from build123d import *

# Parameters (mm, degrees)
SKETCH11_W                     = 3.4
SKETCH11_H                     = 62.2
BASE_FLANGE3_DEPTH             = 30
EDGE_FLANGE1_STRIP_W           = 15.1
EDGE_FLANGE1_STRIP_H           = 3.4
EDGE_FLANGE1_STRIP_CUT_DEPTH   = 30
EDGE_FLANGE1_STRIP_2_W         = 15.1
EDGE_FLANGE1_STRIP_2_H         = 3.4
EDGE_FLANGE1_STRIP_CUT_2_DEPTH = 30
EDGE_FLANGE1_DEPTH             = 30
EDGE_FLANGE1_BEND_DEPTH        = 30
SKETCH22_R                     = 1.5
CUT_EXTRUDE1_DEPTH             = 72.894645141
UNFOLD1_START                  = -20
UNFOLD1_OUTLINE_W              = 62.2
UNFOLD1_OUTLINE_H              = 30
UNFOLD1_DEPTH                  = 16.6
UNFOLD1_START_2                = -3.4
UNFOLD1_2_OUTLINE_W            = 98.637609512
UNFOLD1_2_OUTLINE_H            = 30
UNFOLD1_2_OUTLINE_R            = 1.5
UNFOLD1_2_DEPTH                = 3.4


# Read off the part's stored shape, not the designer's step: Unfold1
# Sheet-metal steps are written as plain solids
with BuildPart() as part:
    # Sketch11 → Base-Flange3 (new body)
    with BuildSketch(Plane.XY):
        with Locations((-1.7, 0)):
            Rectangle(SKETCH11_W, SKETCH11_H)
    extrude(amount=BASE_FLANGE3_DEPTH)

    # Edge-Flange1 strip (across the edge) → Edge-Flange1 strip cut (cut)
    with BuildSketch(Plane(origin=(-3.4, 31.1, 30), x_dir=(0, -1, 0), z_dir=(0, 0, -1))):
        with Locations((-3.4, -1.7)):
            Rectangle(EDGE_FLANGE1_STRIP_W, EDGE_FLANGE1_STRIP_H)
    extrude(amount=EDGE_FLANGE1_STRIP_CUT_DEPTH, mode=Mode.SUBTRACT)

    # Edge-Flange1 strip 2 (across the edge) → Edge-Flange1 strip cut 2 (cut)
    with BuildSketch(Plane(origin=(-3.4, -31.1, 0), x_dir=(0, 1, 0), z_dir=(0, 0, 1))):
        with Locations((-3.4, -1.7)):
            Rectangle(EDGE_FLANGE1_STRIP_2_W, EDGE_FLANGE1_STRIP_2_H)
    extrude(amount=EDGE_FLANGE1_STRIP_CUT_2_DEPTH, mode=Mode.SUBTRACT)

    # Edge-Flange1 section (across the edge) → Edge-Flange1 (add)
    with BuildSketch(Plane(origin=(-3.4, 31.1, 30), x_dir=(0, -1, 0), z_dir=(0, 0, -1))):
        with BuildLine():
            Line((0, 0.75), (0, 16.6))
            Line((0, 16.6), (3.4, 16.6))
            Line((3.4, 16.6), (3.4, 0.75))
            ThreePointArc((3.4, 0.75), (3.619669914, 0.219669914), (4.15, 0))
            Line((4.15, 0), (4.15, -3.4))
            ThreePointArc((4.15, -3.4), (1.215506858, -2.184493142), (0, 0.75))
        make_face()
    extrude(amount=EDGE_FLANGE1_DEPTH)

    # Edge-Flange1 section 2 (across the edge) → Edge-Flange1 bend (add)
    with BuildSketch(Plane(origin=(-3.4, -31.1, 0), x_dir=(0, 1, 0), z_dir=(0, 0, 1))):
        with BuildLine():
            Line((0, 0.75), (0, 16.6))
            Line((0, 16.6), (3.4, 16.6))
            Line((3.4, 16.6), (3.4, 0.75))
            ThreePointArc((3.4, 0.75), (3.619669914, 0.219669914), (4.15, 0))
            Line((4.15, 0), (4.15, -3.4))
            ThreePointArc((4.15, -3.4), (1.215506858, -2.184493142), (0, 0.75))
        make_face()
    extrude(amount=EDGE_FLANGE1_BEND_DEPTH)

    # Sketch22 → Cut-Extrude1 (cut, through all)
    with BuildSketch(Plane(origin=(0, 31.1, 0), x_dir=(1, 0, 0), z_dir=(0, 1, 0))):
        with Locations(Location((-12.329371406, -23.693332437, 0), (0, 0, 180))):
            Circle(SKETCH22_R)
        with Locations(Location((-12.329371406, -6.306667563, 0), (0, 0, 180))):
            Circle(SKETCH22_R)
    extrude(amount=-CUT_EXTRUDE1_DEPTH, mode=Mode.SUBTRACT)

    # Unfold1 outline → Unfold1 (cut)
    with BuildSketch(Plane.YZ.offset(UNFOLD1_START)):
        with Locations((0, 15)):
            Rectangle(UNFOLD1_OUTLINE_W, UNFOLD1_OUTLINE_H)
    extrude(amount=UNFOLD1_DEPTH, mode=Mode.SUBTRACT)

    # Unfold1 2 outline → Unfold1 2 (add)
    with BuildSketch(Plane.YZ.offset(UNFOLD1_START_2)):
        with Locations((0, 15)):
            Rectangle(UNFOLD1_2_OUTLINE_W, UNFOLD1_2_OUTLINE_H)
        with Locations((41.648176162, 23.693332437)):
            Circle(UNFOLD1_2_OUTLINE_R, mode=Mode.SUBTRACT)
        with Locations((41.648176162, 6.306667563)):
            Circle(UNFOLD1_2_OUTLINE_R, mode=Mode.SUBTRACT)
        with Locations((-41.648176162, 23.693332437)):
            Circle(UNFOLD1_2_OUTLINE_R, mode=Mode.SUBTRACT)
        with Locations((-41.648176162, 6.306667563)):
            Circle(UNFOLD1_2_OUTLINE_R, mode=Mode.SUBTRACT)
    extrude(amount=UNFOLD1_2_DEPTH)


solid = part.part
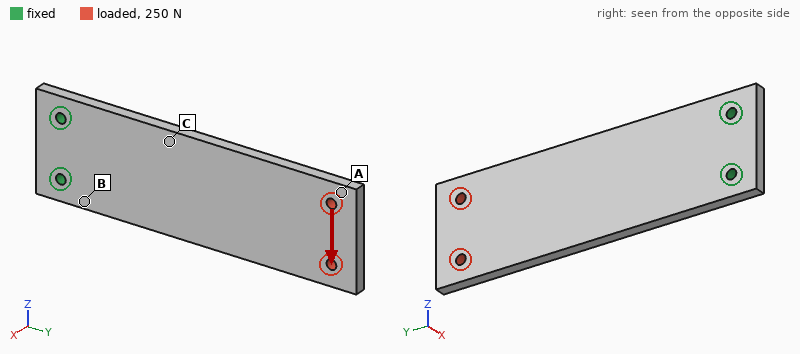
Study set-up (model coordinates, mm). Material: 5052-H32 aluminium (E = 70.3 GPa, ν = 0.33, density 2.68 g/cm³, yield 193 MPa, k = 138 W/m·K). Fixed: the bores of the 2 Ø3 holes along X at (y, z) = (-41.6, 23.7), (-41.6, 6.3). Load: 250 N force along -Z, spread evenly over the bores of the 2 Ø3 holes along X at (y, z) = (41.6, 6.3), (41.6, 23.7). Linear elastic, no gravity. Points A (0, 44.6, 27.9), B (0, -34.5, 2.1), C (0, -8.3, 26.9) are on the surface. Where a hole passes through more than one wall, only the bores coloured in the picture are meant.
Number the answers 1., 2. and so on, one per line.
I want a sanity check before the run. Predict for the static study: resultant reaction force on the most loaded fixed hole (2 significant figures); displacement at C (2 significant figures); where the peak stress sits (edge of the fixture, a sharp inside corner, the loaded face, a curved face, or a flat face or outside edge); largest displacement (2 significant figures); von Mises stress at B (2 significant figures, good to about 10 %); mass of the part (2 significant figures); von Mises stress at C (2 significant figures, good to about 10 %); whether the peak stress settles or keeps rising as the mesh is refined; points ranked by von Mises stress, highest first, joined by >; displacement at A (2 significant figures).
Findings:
1. 1.1 kN
2. 0.030 mm
3. edge of the fixture
4. 0.13 mm
5. 29 MPa
6. 27 g
7. 20 MPa
8. keeps rising
9. B > C > A
10. 0.12 mm
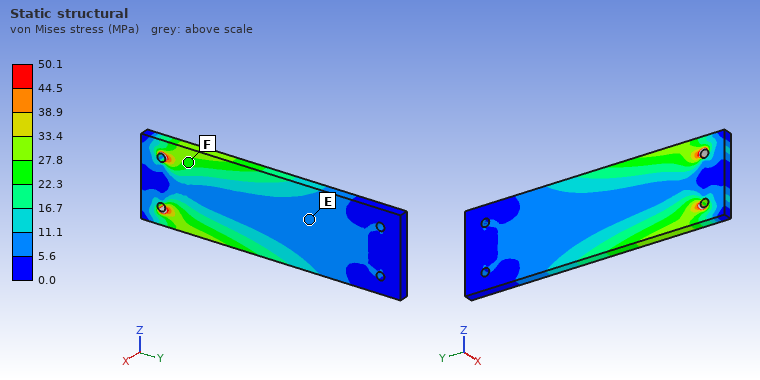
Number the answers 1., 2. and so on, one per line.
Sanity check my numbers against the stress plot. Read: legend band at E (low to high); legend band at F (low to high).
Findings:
1. 5.6 to 11.1 MPa
2. 22.3 to 27.8 MPa
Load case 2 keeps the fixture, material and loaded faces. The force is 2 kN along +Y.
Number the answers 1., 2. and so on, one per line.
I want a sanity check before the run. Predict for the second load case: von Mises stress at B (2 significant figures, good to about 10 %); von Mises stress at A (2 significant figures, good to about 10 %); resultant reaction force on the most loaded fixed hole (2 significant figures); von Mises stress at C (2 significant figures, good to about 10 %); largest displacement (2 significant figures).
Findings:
1. 19 MPa
2. 9.6 MPa
3. 1.0 kN
4. 20 MPa
5. 26 µm
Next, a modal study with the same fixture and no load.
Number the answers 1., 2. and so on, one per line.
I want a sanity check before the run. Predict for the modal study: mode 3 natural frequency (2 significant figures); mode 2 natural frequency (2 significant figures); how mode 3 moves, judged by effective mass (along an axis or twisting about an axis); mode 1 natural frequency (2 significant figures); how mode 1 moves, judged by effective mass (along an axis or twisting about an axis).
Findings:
1. 2100 Hz
2. 2100 Hz
3. along X
4. 340 Hz
5. along X
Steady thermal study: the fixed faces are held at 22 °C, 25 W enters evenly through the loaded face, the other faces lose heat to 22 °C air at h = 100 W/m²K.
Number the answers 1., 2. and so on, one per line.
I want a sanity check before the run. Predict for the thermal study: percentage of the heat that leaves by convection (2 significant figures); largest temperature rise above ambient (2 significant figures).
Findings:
1. 74 %
2. 70 K
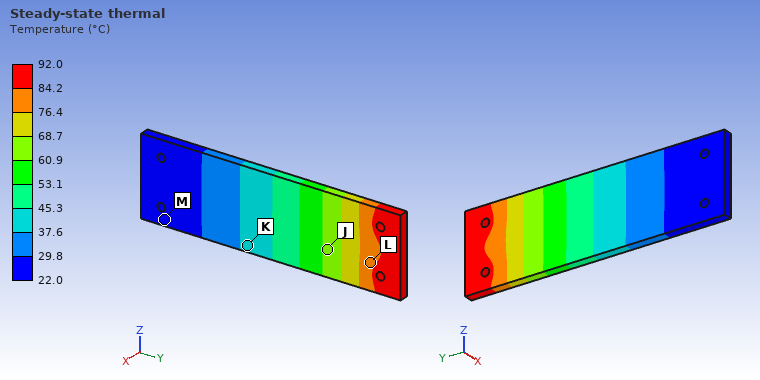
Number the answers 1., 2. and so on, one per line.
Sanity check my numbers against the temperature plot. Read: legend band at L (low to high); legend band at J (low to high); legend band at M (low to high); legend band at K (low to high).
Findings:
1. 76.4 to 84.2 °C
2. 60.9 to 68.7 °C
3. 22.0 to 29.8 °C
4. 37.6 to 45.3 °C
